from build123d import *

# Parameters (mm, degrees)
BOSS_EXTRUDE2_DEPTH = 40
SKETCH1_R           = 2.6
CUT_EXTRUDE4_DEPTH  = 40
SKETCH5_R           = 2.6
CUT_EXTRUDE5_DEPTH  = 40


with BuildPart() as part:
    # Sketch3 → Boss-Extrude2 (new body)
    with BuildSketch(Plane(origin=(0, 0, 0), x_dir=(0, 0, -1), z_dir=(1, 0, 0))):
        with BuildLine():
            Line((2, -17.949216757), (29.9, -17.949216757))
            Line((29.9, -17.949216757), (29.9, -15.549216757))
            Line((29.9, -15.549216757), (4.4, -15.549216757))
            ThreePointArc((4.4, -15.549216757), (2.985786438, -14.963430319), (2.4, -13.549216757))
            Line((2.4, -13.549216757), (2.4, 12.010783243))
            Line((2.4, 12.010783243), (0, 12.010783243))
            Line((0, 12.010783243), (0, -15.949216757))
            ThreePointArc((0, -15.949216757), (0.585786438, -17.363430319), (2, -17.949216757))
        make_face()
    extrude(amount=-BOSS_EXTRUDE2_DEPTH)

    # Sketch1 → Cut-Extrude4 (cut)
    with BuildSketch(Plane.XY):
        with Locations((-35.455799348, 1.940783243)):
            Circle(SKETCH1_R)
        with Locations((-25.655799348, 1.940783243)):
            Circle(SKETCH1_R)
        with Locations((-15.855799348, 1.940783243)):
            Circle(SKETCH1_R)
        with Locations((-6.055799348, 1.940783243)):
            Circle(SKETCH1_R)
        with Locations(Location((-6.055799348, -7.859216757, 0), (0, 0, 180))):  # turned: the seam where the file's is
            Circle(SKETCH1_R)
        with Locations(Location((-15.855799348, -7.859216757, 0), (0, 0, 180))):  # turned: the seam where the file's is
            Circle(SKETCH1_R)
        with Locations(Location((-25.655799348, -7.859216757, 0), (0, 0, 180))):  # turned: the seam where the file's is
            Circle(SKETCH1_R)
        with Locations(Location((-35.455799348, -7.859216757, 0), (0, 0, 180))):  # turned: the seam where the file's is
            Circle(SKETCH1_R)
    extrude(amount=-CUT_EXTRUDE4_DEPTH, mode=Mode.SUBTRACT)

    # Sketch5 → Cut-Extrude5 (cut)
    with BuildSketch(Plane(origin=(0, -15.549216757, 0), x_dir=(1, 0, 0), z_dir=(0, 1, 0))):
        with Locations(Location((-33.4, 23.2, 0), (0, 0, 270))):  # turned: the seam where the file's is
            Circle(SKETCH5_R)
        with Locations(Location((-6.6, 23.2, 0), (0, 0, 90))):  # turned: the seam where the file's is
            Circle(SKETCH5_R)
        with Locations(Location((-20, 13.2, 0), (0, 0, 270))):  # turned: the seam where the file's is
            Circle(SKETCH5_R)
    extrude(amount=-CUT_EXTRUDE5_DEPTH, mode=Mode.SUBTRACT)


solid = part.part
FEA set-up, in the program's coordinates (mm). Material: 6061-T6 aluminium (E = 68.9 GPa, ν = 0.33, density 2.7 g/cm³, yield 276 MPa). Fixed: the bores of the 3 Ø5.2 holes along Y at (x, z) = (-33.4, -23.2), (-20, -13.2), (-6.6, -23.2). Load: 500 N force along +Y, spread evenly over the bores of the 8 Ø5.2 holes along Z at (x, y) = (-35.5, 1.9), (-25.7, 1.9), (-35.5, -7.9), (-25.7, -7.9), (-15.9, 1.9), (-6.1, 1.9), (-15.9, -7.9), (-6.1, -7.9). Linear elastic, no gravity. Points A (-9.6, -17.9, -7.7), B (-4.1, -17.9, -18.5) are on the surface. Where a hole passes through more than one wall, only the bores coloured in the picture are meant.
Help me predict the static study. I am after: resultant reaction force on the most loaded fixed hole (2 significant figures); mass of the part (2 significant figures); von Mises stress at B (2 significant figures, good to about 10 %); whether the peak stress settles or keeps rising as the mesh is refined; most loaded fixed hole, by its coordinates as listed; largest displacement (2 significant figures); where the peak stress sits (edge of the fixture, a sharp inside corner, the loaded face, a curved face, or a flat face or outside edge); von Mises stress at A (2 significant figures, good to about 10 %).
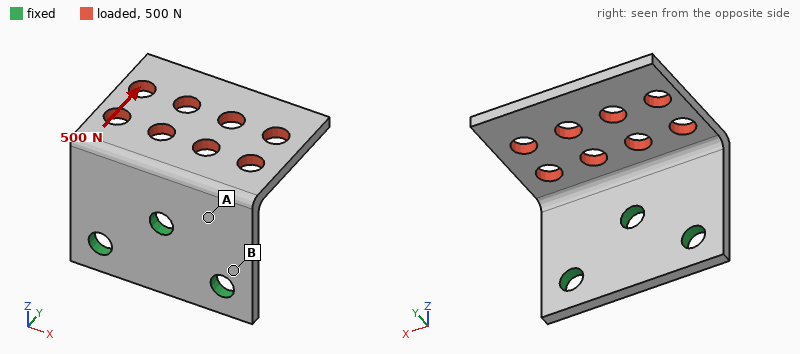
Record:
600 N
13 g
27 MPa
keeps rising
(-20, -13.2)
0.34 mm
edge of the fixture
62 MPa
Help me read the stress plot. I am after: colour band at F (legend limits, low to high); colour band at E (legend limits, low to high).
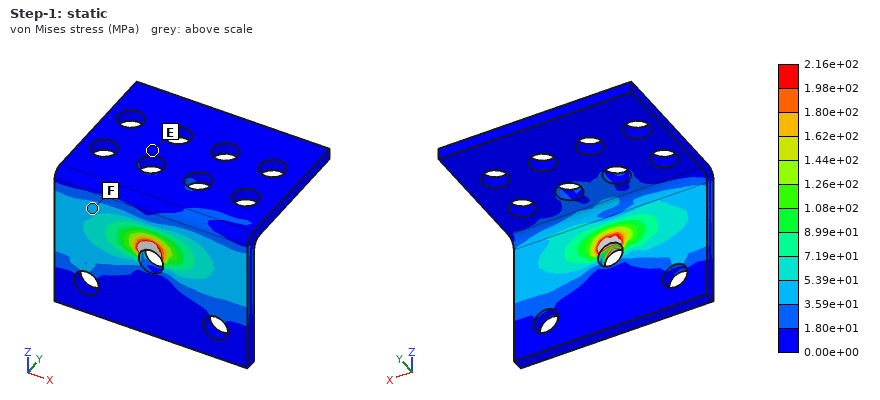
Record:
3.59e+01 to 5.39e+01 MPa
0.00e+00 to 1.80e+01 MPa
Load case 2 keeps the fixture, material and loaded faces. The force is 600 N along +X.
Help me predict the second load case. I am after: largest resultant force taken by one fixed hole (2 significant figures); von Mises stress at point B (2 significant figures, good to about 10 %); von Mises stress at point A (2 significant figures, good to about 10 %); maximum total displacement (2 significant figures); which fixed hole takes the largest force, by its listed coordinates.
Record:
540 N
120 MPa
55 MPa
0.44 mm
(-20, -13.2)
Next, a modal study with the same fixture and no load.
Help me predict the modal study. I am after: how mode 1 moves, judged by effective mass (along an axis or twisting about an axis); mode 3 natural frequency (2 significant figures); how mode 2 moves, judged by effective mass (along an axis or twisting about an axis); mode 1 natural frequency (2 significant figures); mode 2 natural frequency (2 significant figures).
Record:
along Z
4100 Hz
along X
1500 Hz
2400 Hz
